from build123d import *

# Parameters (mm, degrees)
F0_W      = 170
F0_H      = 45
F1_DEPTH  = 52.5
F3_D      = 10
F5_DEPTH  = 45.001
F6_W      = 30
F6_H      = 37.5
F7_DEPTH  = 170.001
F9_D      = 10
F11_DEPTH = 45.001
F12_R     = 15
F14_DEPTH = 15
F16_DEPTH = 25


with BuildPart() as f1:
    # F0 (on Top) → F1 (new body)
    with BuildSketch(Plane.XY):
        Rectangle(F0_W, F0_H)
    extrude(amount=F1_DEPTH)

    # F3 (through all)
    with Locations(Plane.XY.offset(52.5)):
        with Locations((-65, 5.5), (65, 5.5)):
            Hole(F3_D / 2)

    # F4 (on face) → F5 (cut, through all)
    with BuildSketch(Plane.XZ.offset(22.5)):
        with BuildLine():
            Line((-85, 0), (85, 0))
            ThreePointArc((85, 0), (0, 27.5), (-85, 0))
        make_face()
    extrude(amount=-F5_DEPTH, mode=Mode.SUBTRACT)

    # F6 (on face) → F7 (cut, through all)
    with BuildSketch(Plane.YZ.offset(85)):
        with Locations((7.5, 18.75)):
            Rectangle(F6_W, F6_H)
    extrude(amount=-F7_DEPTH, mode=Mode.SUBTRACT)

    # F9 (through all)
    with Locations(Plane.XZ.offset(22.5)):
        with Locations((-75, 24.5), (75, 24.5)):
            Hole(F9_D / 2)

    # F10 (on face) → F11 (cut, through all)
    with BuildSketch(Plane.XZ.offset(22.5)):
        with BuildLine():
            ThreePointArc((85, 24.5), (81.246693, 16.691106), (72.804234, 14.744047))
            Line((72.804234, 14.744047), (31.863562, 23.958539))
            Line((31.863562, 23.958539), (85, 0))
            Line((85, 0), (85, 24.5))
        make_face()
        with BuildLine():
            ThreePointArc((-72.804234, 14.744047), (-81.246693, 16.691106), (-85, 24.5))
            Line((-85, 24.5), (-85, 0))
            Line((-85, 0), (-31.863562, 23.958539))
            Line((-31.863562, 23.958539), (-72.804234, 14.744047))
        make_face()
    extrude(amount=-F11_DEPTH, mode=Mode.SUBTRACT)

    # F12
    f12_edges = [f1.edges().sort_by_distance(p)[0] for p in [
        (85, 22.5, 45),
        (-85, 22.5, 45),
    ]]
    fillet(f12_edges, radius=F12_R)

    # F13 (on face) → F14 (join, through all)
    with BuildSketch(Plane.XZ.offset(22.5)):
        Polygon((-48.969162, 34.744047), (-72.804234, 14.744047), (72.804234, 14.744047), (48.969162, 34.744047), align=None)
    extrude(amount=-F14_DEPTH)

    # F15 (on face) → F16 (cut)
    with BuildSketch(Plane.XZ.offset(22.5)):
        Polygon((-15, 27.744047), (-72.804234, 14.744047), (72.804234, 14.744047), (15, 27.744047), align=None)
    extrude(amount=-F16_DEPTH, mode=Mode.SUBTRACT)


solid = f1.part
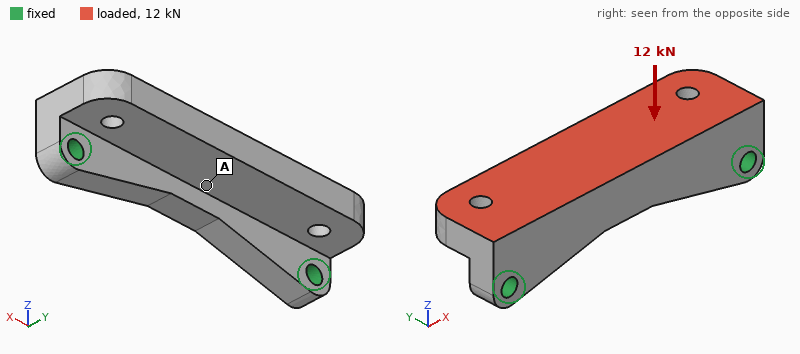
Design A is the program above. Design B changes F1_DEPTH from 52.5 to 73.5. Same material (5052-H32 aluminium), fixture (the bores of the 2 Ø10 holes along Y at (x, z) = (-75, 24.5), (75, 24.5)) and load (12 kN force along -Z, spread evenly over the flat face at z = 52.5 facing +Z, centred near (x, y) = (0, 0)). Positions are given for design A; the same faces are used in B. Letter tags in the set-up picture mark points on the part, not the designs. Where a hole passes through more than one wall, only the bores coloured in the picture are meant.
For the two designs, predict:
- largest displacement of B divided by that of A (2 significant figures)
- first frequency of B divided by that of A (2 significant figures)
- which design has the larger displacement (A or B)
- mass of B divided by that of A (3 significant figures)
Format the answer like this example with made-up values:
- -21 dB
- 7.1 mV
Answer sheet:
- 0.77
- 0.57
- A
- 2.04
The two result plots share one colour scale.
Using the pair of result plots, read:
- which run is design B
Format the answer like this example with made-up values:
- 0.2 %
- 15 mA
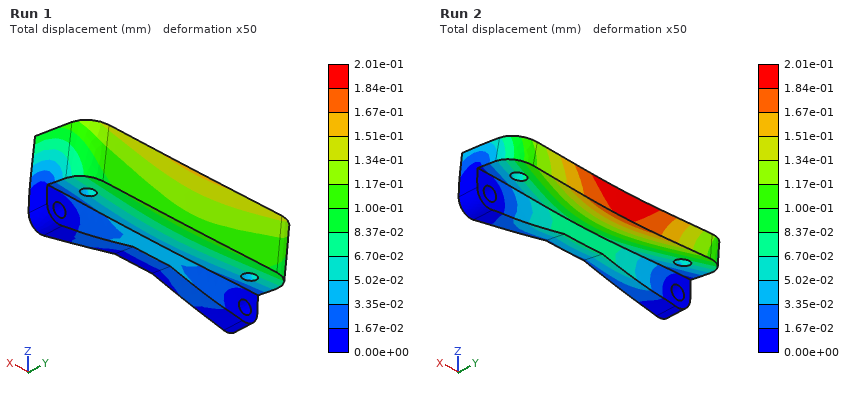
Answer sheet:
- Run 1
